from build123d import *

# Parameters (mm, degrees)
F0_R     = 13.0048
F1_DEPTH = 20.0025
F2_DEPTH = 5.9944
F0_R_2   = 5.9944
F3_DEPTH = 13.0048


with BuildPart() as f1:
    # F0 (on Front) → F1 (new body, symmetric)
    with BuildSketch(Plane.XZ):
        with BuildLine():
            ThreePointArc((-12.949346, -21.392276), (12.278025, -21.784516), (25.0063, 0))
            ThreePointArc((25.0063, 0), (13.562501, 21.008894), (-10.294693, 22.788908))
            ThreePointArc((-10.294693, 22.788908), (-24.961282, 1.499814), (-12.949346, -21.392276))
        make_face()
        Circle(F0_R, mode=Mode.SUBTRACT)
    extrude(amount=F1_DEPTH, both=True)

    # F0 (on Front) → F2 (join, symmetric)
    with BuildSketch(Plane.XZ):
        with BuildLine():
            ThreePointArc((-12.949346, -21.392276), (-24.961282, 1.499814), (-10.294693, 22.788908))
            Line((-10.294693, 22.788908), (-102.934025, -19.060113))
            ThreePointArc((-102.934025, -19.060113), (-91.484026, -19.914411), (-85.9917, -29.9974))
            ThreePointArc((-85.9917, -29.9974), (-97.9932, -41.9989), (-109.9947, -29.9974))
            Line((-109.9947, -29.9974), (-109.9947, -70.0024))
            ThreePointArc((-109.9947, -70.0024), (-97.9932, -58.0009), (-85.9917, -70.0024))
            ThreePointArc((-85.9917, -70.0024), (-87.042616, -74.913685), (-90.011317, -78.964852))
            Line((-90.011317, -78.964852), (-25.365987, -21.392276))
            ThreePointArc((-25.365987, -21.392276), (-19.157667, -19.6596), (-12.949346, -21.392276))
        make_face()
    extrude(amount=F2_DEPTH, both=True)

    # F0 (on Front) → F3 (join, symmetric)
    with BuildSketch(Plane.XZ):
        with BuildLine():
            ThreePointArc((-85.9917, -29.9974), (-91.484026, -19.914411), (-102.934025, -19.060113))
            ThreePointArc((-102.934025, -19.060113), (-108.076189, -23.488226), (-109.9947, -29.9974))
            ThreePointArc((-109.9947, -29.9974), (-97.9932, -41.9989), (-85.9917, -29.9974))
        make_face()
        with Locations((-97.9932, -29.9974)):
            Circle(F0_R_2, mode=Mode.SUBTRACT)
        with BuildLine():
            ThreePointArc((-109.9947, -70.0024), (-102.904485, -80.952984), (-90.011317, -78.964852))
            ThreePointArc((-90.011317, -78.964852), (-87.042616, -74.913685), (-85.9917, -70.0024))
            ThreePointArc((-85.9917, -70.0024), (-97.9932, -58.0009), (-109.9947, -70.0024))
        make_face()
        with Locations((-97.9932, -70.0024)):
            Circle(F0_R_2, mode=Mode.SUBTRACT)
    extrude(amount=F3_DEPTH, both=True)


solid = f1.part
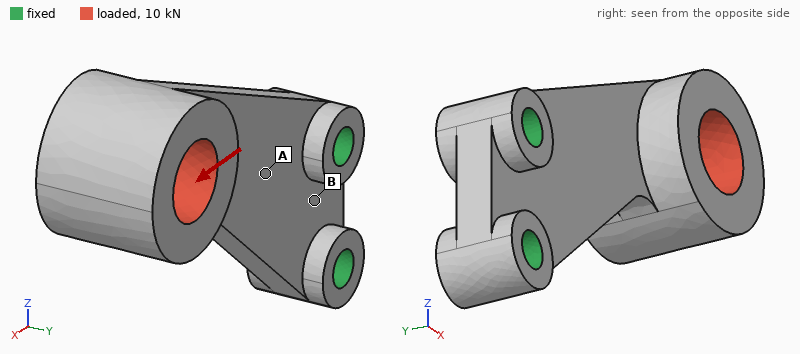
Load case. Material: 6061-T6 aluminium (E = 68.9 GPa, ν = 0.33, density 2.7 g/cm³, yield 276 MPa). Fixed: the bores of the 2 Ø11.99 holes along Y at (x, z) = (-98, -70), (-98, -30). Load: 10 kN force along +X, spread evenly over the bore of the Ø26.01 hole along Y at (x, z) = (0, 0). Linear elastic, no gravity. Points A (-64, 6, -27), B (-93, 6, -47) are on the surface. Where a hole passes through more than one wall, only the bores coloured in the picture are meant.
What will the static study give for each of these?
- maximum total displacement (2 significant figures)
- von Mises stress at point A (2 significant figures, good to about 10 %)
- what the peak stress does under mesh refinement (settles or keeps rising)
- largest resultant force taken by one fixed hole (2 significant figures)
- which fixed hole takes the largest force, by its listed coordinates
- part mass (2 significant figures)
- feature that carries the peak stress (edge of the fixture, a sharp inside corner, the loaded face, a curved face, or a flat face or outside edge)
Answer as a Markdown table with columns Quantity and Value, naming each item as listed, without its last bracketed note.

| Quantity | Value |
|---|---|
| maximum total displacement | 0.29 mm |
| von Mises stress at point A | 23 MPa |
| what the peak stress does under mesh refinement | keeps rising |
| largest resultant force taken by one fixed hole | 16 kN |
| which fixed hole takes the largest force, by its listed coordinates | (-98, -30) |
| part mass | 320 g |
| feature that carries the peak stress | edge of the fixture |
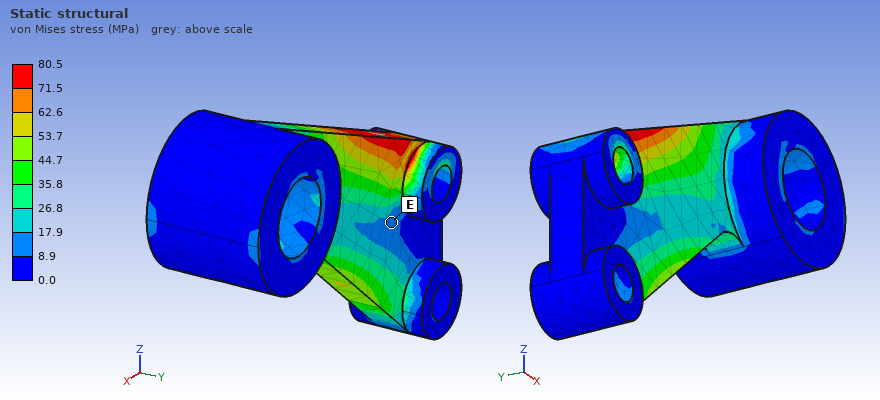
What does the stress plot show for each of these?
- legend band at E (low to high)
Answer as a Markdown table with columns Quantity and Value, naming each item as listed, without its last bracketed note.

| Quantity | Value |
|---|---|
| legend band at E | 8.9 to 17.9 MPa |
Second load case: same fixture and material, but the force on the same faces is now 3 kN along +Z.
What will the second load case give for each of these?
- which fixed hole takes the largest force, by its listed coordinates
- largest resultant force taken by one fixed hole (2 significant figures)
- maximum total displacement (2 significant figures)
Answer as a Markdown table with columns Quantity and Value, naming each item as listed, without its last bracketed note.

| Quantity | Value |
|---|---|
| which fixed hole takes the largest force, by its listed coordinates | (-98, -70) |
| largest resultant force taken by one fixed hole | 7.1 kN |
| maximum total displacement | 0.25 mm |
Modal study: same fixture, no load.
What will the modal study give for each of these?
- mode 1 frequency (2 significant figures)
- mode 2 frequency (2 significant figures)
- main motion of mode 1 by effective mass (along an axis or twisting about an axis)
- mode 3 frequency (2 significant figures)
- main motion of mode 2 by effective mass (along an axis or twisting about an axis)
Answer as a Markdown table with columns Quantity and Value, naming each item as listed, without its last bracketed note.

| Quantity | Value |
|---|---|
| mode 1 frequency | 460 Hz |
| mode 2 frequency | 1500 Hz |
| main motion of mode 1 by effective mass | along Y |
| mode 3 frequency | 1800 Hz |
| main motion of mode 2 by effective mass | along Z |
